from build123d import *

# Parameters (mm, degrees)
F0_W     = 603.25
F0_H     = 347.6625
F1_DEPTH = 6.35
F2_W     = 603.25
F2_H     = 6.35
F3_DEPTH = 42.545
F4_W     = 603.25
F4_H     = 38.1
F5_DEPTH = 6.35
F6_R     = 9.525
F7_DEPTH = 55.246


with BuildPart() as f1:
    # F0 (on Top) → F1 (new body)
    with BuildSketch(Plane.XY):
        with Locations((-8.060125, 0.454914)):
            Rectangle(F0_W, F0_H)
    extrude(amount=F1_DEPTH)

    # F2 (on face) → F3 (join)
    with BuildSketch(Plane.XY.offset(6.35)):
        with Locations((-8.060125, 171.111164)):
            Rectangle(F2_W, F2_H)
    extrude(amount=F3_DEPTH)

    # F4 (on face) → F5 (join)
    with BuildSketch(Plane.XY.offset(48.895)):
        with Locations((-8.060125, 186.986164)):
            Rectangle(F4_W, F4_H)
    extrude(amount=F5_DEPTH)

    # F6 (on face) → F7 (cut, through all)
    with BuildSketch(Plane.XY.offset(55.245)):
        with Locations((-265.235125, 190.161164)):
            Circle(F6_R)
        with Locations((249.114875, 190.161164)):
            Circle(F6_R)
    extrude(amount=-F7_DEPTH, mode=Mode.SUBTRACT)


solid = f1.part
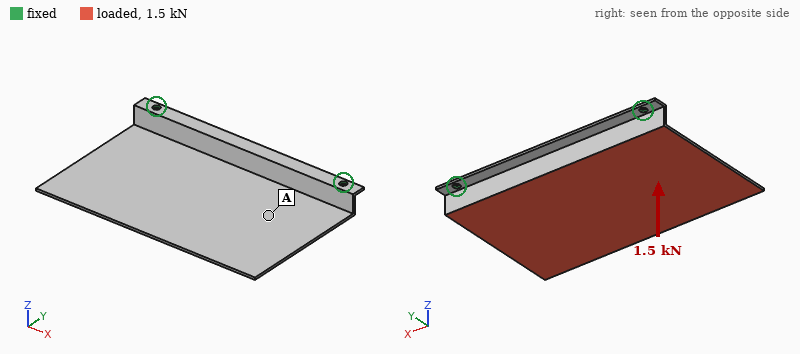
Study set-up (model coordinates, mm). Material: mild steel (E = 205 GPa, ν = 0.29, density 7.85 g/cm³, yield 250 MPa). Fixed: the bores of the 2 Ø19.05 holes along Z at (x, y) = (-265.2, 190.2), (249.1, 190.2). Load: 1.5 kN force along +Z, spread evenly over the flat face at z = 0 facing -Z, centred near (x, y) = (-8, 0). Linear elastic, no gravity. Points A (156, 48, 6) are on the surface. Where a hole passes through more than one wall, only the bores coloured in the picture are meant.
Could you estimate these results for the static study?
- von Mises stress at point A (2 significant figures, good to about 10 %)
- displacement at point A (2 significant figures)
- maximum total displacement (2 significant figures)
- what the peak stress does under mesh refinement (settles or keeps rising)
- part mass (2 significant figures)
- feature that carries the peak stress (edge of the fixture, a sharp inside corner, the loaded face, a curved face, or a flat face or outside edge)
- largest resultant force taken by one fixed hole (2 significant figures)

24 MPa
2.0 mm
6.8 mm
keeps rising
13 kg
edge of the fixture
2.4 kN
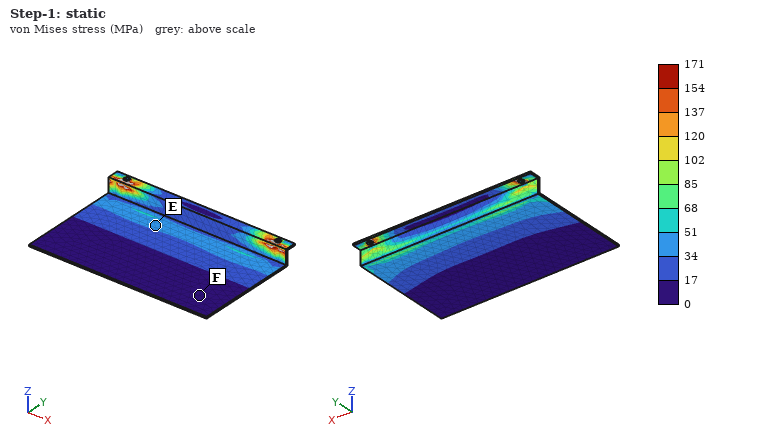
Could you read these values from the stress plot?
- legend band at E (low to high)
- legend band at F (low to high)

34 to 51 MPa
0 to 17 MPa
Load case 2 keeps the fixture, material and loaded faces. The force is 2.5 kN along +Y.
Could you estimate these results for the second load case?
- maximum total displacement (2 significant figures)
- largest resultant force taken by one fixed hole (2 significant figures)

1.7 mm
1.3 kN
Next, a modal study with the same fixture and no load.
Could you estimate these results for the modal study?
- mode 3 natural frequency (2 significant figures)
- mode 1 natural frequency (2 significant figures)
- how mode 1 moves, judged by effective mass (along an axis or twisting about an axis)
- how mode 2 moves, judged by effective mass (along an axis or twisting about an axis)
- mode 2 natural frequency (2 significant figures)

150 Hz
28 Hz
along Z
twisting about Y
64 Hz
